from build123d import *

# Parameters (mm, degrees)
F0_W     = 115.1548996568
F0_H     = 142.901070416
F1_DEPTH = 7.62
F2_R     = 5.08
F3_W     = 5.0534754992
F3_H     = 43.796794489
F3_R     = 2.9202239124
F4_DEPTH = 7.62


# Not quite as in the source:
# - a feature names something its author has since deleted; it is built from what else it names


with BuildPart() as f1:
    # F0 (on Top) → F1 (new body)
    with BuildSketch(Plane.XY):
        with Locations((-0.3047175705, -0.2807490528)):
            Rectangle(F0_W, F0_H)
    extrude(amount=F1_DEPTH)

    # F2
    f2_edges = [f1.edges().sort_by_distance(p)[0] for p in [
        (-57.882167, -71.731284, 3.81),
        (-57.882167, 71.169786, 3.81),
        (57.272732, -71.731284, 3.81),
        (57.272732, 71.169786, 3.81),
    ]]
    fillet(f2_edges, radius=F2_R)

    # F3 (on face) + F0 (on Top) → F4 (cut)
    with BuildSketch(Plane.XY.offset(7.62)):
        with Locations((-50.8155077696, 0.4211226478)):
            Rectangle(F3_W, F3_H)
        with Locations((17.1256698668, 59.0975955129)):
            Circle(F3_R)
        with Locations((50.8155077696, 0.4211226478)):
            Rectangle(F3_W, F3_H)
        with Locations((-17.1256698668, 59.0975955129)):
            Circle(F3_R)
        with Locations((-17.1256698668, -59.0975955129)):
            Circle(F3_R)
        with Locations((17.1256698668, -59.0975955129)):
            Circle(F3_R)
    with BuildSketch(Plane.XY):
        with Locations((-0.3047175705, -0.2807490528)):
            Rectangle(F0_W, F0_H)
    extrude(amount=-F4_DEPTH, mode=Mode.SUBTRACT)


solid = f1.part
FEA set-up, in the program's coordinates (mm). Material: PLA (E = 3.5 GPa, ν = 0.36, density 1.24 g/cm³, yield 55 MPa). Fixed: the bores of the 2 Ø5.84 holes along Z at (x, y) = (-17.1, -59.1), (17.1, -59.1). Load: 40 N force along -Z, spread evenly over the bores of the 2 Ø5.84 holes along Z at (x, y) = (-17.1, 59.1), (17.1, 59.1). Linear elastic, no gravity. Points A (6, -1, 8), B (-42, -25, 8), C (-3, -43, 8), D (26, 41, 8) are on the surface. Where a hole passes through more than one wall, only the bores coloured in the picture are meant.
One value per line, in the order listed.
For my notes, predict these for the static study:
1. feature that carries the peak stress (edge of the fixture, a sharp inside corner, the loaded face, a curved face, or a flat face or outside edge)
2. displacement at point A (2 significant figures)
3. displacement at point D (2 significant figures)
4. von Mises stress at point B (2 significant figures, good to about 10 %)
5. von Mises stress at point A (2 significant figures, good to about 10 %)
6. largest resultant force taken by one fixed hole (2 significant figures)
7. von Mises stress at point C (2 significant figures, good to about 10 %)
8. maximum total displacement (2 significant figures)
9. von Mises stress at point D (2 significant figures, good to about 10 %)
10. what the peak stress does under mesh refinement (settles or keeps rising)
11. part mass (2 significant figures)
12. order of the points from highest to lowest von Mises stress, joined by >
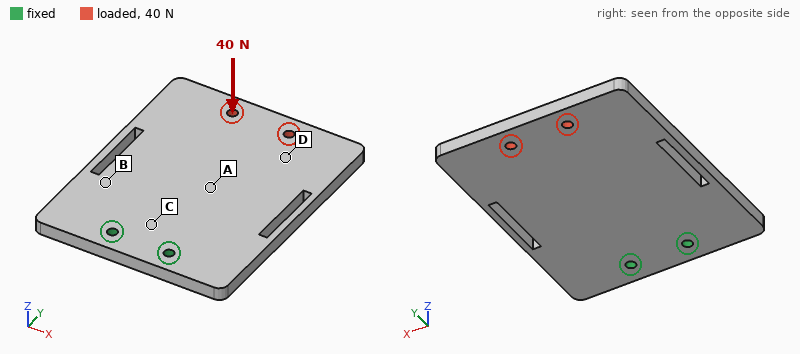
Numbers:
edge of the fixture
0.58 mm
1.4 mm
2.9 MPa
2.1 MPa
20 N
4.1 MPa
2.0 mm
0.86 MPa
keeps rising
150 g
C > B > A > D
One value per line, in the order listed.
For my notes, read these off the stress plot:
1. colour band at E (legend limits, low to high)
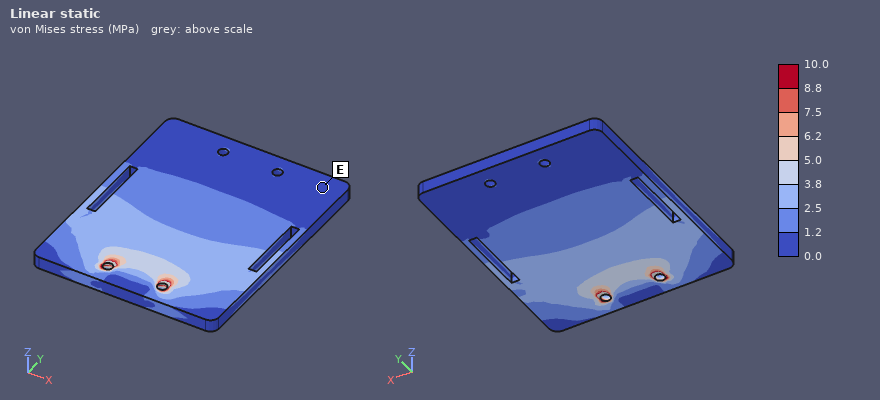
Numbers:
0.0 to 1.2 MPa
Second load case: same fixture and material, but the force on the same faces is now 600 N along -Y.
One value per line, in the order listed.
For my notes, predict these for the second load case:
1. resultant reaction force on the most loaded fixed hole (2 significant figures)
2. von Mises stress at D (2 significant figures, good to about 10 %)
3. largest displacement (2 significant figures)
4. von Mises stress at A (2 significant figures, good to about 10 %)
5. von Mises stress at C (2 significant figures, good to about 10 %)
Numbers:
300 N
1.0 MPa
43 µm
1.1 MPa
0.88 MPa
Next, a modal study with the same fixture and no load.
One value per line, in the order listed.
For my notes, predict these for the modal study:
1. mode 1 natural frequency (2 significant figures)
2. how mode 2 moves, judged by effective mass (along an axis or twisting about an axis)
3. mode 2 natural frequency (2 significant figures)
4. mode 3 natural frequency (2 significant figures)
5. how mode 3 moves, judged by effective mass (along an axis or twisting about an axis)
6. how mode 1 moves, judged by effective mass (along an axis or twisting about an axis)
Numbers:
110 Hz
twisting about Y
270 Hz
620 Hz
along X
along Z
